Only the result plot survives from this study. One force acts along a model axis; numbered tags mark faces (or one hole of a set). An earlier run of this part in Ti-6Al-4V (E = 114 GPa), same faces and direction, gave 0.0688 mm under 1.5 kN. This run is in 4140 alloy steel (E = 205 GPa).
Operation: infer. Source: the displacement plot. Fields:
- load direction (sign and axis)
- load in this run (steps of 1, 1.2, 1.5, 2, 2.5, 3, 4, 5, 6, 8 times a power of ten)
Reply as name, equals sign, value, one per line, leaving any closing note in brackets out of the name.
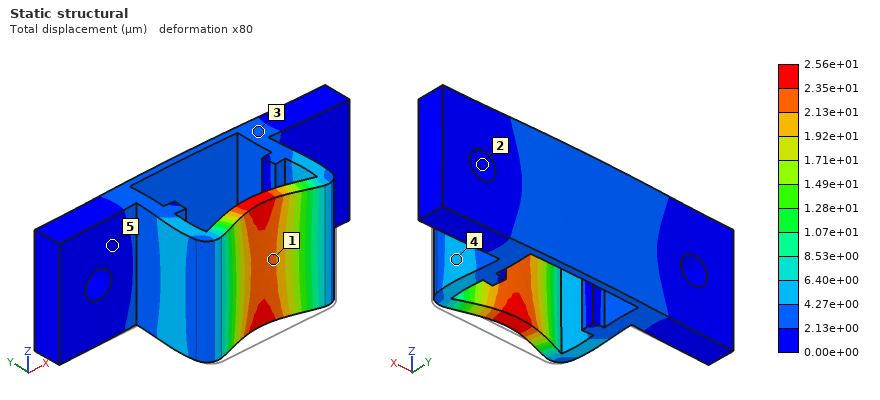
load direction = +Y
load in this run = 1 kN
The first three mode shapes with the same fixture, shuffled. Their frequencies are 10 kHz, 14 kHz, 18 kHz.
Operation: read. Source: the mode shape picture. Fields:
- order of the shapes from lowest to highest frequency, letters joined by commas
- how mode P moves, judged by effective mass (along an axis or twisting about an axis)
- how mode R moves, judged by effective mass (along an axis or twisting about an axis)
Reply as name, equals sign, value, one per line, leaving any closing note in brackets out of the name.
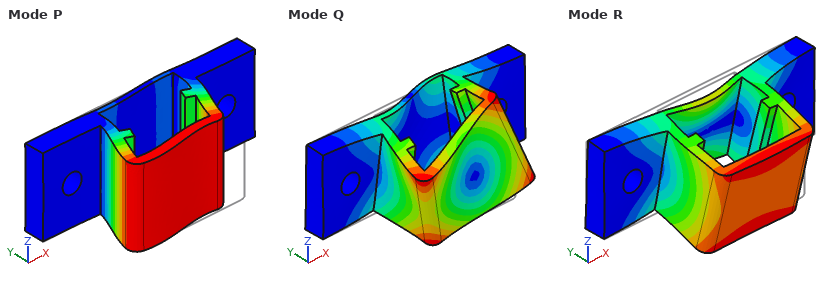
order of the shapes from lowest to highest frequency, letters joined by commas = P, R, Q
how mode P moves, judged by effective mass = along X
how mode R moves, judged by effective mass = along Z
